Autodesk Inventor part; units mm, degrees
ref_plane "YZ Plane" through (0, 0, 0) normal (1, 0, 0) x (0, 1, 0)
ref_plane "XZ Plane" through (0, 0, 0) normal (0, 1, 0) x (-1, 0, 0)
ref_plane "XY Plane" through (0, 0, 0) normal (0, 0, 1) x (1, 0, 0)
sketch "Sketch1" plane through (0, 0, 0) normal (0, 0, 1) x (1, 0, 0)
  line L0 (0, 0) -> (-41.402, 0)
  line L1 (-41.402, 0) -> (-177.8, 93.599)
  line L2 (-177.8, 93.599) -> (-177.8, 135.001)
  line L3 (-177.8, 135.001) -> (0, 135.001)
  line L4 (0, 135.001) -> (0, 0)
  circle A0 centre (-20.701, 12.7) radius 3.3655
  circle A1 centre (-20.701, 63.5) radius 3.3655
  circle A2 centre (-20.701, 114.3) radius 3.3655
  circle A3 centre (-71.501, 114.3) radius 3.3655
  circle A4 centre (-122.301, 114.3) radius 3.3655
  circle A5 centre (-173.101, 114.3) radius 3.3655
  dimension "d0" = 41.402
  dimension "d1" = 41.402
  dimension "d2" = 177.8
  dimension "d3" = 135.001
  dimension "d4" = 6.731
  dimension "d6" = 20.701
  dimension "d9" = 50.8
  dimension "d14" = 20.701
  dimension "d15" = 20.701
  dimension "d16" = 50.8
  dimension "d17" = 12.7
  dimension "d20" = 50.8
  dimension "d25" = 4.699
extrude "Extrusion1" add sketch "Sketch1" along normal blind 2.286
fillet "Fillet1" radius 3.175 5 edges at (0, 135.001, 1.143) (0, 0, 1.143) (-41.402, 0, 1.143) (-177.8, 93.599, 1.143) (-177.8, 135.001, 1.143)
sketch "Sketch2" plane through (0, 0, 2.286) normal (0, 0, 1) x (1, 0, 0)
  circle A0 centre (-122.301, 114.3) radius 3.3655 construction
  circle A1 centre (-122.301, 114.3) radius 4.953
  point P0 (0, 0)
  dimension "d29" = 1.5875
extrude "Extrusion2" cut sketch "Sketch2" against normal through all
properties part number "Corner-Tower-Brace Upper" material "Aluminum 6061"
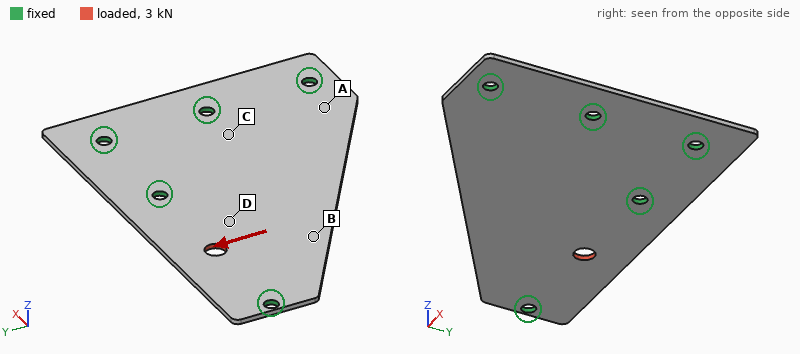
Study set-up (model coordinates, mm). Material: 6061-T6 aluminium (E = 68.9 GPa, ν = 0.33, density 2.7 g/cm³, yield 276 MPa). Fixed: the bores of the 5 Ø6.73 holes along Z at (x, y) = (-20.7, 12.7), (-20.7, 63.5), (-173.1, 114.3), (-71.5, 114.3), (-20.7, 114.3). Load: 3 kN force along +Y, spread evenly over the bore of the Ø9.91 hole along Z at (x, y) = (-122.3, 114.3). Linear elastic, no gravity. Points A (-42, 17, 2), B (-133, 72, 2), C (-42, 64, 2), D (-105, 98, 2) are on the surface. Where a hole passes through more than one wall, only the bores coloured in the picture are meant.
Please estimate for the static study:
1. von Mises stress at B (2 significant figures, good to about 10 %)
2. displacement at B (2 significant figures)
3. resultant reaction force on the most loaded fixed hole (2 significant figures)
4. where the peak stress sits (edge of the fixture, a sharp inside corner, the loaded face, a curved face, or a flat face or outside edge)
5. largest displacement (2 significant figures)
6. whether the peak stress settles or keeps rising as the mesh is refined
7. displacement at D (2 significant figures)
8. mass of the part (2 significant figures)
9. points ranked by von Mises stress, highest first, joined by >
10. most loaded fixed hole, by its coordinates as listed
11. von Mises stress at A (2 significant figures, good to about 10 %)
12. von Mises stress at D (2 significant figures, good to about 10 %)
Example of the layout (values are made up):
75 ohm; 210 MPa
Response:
16 MPa; 24 µm; 1.6 kN; edge of the fixture; 39 µm; keeps rising; 21 µm; 110 g; D > B > A > C; (-71.5, 114.3); 7.9 MPa; 28 MPa
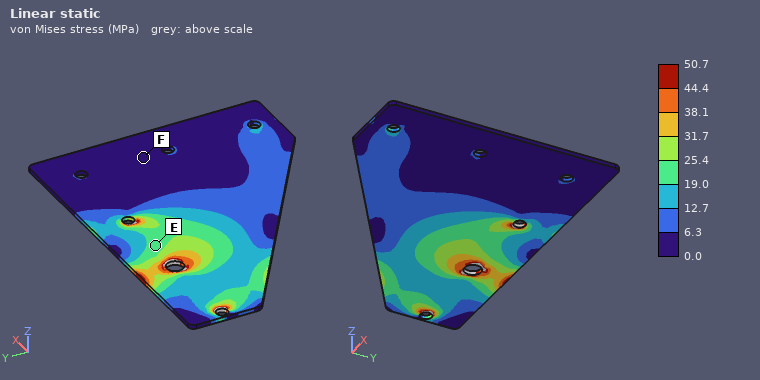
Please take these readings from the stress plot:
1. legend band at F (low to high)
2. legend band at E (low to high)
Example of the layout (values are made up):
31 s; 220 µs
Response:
0.0 to 6.3 MPa; 19.0 to 25.4 MPa
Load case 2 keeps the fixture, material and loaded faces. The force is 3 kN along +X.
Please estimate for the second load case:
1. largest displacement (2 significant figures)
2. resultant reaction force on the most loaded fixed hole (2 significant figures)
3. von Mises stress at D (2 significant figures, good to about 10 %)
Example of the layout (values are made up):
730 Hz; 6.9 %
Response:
18 µm; 1.2 kN; 12 MPa
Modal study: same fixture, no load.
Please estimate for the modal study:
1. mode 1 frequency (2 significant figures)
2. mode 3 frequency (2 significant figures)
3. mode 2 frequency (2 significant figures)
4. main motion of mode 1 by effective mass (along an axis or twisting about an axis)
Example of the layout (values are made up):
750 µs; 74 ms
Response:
550 Hz; 1400 Hz; 1100 Hz; along Z
